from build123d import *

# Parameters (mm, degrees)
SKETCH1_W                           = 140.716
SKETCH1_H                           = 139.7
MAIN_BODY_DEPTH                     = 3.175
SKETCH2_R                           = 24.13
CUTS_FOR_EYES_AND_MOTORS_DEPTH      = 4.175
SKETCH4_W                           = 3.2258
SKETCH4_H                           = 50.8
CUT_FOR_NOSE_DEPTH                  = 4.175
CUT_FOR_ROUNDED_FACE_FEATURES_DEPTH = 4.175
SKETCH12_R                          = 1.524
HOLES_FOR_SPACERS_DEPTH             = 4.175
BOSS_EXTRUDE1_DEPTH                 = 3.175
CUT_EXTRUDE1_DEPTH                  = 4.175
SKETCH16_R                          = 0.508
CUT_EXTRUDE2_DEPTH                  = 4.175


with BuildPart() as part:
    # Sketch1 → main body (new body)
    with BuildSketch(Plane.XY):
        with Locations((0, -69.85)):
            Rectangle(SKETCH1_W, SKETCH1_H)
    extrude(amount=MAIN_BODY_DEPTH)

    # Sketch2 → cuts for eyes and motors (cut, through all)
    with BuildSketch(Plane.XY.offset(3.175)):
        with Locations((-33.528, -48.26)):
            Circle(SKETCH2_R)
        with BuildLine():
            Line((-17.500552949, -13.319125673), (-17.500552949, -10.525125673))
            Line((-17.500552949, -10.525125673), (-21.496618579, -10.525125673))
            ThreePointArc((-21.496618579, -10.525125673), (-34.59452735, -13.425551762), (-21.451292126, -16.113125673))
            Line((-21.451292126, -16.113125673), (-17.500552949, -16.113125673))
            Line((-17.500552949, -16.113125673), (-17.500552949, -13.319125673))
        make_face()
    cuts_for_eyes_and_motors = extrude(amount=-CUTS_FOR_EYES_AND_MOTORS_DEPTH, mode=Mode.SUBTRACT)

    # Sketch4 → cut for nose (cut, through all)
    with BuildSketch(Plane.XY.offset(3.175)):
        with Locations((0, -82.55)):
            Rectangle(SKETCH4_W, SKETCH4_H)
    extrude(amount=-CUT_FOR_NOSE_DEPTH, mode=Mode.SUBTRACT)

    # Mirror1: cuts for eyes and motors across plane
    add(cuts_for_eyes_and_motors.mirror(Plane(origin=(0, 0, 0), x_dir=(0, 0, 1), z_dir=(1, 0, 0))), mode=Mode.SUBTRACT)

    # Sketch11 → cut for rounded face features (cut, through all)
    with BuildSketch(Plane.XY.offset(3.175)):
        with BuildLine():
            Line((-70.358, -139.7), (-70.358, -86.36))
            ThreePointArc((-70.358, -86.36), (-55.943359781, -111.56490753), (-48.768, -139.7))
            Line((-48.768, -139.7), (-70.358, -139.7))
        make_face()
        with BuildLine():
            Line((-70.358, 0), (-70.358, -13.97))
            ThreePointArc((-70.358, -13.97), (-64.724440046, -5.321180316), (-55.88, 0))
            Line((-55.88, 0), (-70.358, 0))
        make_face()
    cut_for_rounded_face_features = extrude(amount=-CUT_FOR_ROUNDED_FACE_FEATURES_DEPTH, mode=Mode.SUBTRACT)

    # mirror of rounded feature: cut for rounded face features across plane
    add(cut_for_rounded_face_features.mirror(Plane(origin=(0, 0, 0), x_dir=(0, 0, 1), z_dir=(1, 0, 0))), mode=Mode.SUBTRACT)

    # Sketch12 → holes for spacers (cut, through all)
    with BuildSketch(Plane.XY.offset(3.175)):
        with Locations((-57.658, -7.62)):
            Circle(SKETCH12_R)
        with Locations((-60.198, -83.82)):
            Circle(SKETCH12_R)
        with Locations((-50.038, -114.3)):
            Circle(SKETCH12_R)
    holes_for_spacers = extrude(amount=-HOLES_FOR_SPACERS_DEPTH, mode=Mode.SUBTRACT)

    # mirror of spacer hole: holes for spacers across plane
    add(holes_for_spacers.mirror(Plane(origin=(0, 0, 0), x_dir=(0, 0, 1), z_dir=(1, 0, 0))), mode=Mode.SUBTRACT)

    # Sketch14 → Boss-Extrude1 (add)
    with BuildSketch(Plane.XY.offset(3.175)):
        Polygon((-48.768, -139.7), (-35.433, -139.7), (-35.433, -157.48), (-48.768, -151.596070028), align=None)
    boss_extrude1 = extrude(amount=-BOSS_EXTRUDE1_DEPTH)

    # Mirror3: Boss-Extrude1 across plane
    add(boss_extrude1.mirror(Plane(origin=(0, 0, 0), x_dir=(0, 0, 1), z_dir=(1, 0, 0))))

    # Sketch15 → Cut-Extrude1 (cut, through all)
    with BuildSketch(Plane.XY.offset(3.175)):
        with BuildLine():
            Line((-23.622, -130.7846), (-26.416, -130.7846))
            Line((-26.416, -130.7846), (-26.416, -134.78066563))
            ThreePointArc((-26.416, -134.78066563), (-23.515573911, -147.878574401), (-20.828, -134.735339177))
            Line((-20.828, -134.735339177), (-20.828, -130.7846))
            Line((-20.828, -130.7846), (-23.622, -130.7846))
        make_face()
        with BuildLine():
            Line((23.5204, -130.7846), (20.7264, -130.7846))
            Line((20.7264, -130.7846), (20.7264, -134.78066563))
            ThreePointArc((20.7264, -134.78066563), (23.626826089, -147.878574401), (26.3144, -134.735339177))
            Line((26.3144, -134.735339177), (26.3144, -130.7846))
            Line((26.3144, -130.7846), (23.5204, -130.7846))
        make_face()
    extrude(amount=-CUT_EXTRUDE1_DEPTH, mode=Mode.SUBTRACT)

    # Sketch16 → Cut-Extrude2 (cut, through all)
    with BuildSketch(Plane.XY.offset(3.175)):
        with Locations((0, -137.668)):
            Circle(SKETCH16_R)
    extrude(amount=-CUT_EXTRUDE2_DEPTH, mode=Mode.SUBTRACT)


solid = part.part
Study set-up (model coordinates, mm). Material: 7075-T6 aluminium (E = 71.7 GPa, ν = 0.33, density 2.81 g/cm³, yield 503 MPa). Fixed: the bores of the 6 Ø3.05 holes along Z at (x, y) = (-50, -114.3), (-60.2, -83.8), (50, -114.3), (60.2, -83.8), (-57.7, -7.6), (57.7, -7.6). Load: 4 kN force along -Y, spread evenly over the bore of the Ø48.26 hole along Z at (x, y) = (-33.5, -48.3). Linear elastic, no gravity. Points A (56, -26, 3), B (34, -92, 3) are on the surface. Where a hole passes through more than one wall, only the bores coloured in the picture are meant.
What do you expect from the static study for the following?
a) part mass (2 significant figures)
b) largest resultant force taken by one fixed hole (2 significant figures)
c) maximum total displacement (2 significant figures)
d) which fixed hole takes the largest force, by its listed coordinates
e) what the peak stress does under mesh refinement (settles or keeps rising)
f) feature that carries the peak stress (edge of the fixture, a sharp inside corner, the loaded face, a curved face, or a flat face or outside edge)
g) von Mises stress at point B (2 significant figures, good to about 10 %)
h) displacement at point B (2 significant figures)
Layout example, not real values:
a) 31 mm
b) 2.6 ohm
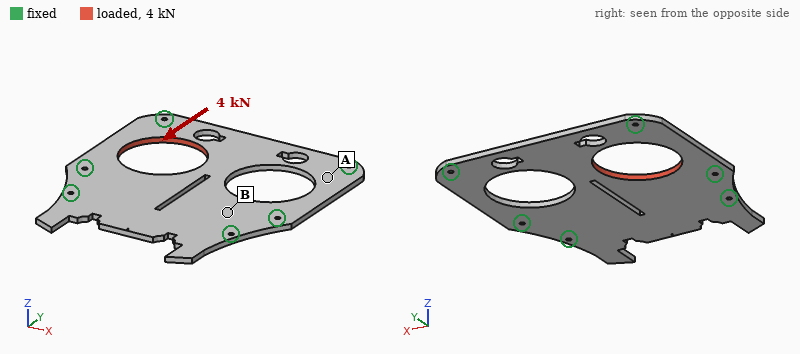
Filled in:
a) 130 g
b) 1.2 kN
c) 26 µm
d) (-57.7, -7.6)
e) keeps rising
f) edge of the fixture
g) 9.8 MPa
h) 5.5 µm
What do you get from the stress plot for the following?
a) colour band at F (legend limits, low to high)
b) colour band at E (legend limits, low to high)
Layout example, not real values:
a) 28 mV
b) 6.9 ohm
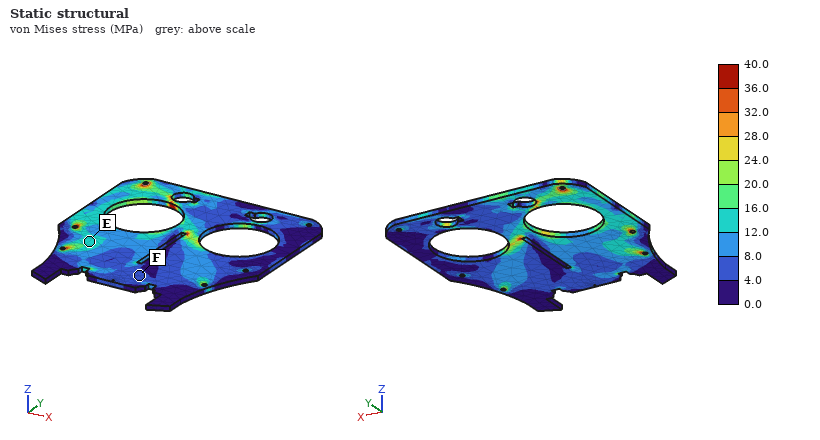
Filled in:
a) 4.0 to 8.0 MPa
b) 12.0 to 16.0 MPa
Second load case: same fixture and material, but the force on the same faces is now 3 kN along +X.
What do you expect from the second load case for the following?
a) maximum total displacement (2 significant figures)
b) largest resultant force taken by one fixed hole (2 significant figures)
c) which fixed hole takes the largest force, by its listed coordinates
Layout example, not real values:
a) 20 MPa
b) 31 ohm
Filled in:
a) 25 µm
b) 1.2 kN
c) (-60.2, -83.8)
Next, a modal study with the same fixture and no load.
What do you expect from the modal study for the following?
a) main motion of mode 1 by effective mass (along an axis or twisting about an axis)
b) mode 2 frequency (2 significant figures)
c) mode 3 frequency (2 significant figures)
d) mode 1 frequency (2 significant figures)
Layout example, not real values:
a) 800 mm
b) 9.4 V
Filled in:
a) along Z
b) 1300 Hz
c) 1500 Hz
d) 1000 Hz
